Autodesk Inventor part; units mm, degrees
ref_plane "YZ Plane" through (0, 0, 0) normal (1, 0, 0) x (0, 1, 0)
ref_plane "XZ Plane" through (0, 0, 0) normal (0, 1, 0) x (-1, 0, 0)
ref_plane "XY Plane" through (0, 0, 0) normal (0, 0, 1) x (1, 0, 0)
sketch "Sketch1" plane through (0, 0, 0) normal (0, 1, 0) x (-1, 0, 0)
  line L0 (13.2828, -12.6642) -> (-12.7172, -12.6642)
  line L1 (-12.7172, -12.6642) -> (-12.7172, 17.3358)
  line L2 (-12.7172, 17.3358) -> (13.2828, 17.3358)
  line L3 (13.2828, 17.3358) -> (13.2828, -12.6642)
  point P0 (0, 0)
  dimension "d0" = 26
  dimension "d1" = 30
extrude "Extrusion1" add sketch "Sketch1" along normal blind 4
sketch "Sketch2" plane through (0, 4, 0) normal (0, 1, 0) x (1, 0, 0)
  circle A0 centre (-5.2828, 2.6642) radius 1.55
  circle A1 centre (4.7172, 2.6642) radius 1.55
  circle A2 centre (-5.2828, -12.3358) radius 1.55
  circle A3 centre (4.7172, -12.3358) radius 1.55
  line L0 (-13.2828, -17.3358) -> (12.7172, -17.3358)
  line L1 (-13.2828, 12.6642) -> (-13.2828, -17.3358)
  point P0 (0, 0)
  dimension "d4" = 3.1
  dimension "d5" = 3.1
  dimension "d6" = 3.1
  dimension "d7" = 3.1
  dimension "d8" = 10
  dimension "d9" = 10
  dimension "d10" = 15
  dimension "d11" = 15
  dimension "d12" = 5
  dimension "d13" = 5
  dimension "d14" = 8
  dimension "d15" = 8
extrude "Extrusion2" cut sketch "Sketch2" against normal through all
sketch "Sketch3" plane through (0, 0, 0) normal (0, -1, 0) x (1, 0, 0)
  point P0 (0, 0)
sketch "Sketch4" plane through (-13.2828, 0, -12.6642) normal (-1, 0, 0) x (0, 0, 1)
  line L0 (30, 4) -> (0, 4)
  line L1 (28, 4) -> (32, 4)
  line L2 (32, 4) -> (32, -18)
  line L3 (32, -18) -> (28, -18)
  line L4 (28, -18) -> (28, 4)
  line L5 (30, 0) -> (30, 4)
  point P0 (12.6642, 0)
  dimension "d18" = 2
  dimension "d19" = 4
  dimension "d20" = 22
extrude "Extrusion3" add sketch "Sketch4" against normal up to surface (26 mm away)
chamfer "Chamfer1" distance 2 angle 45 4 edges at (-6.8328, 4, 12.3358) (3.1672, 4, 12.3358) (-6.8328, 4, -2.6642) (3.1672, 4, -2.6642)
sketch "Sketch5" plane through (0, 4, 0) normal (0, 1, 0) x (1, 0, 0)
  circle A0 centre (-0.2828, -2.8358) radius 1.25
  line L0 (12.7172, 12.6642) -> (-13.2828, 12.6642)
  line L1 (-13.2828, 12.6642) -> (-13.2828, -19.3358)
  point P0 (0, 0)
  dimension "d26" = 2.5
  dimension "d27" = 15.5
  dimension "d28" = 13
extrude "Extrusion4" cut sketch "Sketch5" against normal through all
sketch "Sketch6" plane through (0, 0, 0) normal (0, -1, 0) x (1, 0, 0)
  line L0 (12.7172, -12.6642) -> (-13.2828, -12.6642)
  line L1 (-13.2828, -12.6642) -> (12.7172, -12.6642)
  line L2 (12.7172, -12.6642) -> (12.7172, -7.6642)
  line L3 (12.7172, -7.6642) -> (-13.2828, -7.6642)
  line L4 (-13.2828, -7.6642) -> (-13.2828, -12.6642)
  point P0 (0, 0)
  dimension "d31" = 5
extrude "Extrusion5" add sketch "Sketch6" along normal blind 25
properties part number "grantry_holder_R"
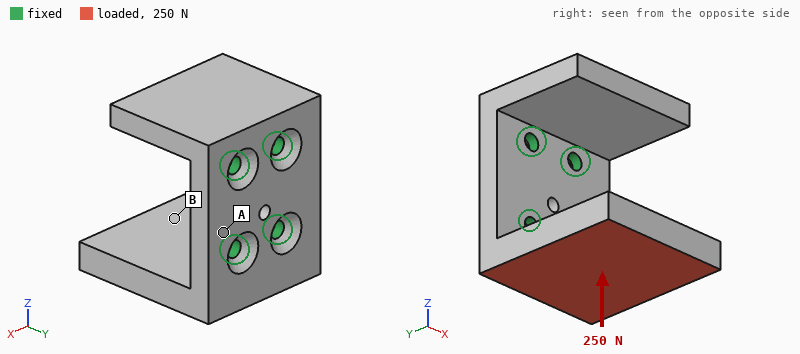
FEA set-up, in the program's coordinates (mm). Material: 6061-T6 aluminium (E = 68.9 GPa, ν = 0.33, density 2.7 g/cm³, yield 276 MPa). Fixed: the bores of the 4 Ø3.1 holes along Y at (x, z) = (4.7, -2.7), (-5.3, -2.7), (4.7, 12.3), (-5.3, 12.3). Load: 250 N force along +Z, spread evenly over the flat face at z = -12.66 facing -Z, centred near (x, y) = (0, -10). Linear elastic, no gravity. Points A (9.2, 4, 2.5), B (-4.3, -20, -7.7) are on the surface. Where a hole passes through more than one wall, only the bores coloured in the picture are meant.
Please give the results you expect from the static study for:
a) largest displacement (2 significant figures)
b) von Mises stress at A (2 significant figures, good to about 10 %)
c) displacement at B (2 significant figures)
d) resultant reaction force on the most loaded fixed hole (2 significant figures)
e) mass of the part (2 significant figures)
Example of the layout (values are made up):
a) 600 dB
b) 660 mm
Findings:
a) 0.11 mm
b) 14 MPa
c) 0.083 mm
d) 220 N
e) 22 g
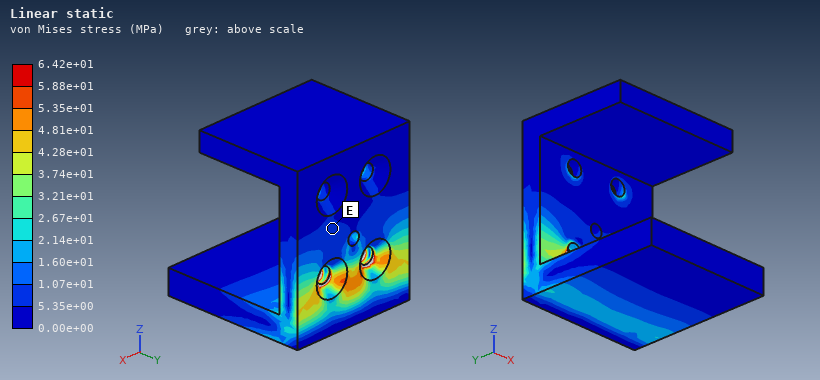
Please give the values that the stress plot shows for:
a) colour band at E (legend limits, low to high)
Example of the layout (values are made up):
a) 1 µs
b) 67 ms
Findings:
a) 5.35e+00 to 1.07e+01 MPa
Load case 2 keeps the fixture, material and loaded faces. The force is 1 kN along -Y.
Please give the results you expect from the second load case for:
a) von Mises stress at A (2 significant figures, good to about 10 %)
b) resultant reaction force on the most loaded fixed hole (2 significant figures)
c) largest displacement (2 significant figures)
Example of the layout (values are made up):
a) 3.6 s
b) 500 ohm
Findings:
a) 45 MPa
b) 740 N
c) 0.23 mm
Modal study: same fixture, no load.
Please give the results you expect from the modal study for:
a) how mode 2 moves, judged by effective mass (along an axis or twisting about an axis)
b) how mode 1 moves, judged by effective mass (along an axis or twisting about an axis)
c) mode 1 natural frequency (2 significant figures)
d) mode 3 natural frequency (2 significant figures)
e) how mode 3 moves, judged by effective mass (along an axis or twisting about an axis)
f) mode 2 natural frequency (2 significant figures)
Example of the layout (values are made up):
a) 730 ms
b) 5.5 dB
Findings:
a) along Z
b) along Z
c) 2900 Hz
d) 5700 Hz
e) along X
f) 5400 Hz
